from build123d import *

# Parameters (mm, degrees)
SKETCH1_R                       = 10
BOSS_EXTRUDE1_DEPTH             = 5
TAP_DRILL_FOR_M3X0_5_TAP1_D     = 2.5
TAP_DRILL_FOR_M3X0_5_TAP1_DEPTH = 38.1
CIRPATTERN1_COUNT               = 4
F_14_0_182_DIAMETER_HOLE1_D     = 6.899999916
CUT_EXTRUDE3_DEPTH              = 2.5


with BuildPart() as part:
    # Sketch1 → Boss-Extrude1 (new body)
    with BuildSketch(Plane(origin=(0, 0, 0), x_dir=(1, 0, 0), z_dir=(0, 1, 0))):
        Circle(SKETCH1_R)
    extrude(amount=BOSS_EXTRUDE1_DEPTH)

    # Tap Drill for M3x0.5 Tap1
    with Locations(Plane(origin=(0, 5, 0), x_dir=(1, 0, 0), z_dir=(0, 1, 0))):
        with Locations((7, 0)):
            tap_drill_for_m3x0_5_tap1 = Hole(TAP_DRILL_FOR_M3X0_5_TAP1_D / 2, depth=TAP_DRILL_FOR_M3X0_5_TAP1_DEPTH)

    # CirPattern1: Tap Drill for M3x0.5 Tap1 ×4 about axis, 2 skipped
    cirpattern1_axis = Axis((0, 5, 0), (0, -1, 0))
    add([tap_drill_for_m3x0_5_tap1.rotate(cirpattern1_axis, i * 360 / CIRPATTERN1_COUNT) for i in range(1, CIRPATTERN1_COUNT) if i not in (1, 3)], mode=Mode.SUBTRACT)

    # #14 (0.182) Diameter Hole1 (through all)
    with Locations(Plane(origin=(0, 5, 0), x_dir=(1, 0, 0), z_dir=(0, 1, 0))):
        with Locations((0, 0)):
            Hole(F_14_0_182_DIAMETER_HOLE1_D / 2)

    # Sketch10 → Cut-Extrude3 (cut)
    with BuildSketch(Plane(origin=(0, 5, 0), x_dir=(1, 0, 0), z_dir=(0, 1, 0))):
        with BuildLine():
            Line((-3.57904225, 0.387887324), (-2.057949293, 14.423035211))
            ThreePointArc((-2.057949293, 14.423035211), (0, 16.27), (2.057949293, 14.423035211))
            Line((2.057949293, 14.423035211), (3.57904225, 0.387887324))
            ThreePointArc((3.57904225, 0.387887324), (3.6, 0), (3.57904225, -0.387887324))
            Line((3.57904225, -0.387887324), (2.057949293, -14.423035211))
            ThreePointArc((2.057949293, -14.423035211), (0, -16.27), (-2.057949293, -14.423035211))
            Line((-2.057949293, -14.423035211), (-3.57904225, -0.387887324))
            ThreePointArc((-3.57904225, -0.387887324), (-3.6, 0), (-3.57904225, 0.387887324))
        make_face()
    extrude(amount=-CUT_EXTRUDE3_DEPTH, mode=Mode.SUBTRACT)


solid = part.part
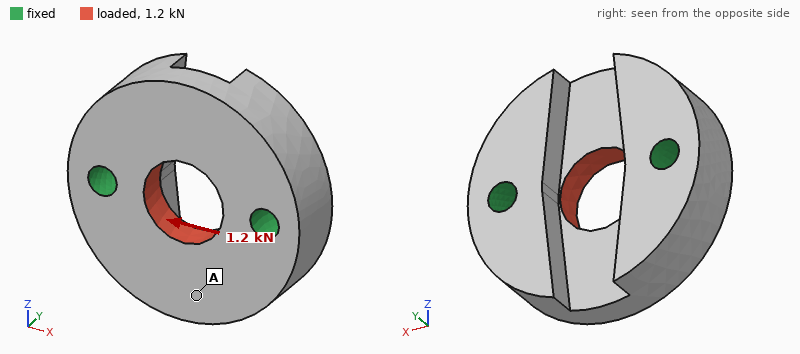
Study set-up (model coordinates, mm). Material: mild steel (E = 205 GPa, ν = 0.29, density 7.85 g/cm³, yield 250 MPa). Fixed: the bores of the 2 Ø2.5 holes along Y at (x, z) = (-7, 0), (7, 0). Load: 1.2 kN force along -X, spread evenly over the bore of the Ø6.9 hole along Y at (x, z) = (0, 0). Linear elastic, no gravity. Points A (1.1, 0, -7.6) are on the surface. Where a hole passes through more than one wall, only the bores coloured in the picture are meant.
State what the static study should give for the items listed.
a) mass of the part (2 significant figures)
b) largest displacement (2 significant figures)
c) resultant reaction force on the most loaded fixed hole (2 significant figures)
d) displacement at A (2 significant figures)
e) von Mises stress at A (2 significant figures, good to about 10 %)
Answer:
8.8 g
0.98 µm
600 N
0.51 µm
8.7 MPa
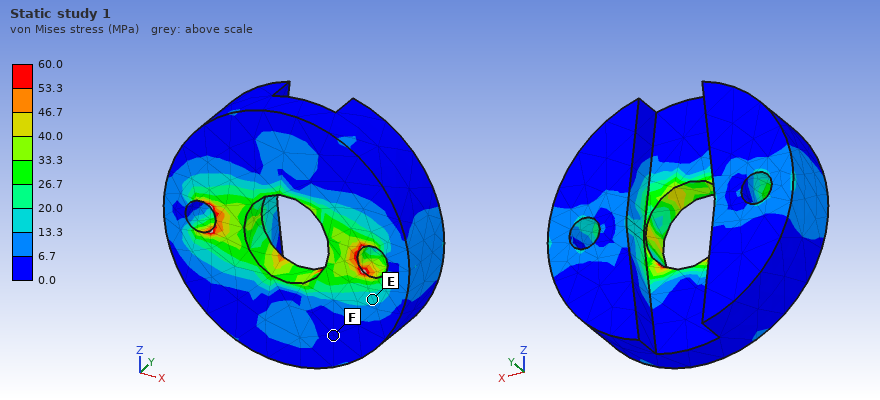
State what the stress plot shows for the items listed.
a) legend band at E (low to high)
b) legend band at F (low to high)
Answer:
13.3 to 20.0 MPa
0.0 to 6.7 MPa
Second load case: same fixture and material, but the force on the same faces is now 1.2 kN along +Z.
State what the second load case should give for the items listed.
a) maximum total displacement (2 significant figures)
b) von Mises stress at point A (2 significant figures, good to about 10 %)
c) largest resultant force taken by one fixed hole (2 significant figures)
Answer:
1.7 µm
11 MPa
600 N
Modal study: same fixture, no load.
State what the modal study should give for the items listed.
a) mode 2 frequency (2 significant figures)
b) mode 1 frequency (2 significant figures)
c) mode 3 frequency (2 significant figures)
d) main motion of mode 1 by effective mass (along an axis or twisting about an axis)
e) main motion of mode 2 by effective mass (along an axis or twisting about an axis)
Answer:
43 kHz
39 kHz
61 kHz
twisting about X
along Y
